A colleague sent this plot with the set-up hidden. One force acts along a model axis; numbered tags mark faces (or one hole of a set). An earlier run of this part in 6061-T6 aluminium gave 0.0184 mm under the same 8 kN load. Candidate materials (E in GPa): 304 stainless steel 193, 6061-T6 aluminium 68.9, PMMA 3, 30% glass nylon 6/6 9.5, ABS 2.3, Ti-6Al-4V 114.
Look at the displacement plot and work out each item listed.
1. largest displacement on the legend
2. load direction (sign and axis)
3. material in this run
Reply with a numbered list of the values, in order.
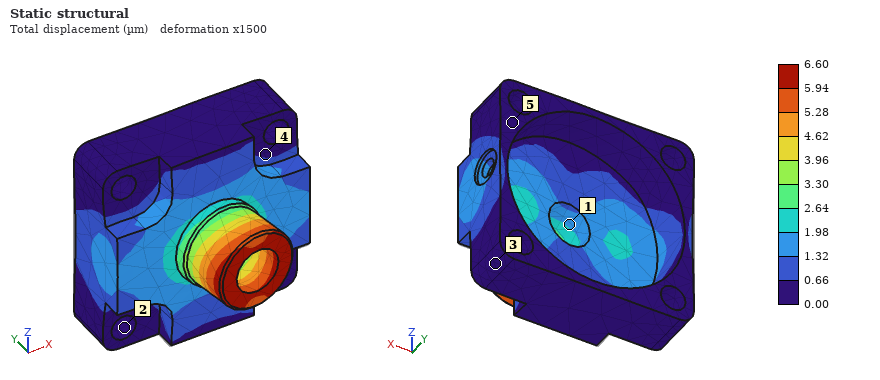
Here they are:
1. 6.60 µm
2. +X
3. 304 stainless steel
